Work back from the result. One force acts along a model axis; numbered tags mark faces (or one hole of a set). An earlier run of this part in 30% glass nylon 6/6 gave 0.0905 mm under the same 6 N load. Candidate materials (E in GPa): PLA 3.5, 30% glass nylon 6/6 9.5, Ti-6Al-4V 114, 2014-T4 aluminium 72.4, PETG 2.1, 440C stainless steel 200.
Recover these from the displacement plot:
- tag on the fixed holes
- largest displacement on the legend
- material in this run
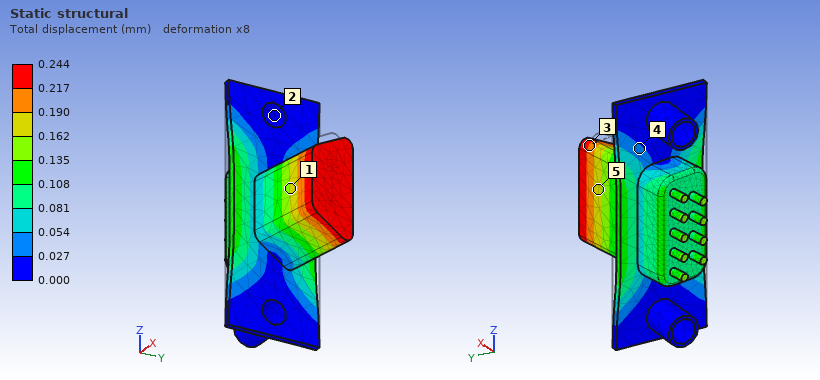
2
0.244 mm
PLA
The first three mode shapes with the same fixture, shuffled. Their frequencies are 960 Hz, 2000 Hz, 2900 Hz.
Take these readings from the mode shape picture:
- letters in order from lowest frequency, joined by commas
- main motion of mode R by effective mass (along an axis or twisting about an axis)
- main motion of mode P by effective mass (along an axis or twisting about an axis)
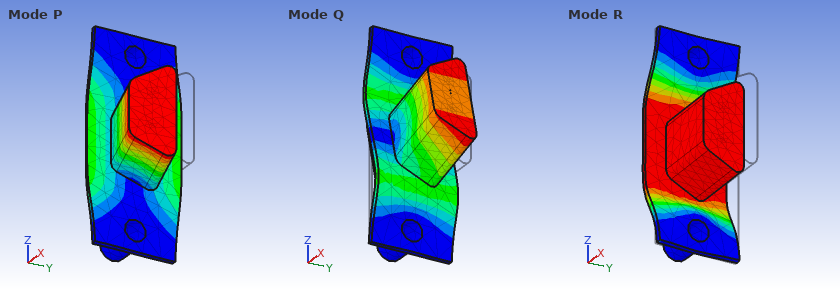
P, R, Q
along X
along Y
